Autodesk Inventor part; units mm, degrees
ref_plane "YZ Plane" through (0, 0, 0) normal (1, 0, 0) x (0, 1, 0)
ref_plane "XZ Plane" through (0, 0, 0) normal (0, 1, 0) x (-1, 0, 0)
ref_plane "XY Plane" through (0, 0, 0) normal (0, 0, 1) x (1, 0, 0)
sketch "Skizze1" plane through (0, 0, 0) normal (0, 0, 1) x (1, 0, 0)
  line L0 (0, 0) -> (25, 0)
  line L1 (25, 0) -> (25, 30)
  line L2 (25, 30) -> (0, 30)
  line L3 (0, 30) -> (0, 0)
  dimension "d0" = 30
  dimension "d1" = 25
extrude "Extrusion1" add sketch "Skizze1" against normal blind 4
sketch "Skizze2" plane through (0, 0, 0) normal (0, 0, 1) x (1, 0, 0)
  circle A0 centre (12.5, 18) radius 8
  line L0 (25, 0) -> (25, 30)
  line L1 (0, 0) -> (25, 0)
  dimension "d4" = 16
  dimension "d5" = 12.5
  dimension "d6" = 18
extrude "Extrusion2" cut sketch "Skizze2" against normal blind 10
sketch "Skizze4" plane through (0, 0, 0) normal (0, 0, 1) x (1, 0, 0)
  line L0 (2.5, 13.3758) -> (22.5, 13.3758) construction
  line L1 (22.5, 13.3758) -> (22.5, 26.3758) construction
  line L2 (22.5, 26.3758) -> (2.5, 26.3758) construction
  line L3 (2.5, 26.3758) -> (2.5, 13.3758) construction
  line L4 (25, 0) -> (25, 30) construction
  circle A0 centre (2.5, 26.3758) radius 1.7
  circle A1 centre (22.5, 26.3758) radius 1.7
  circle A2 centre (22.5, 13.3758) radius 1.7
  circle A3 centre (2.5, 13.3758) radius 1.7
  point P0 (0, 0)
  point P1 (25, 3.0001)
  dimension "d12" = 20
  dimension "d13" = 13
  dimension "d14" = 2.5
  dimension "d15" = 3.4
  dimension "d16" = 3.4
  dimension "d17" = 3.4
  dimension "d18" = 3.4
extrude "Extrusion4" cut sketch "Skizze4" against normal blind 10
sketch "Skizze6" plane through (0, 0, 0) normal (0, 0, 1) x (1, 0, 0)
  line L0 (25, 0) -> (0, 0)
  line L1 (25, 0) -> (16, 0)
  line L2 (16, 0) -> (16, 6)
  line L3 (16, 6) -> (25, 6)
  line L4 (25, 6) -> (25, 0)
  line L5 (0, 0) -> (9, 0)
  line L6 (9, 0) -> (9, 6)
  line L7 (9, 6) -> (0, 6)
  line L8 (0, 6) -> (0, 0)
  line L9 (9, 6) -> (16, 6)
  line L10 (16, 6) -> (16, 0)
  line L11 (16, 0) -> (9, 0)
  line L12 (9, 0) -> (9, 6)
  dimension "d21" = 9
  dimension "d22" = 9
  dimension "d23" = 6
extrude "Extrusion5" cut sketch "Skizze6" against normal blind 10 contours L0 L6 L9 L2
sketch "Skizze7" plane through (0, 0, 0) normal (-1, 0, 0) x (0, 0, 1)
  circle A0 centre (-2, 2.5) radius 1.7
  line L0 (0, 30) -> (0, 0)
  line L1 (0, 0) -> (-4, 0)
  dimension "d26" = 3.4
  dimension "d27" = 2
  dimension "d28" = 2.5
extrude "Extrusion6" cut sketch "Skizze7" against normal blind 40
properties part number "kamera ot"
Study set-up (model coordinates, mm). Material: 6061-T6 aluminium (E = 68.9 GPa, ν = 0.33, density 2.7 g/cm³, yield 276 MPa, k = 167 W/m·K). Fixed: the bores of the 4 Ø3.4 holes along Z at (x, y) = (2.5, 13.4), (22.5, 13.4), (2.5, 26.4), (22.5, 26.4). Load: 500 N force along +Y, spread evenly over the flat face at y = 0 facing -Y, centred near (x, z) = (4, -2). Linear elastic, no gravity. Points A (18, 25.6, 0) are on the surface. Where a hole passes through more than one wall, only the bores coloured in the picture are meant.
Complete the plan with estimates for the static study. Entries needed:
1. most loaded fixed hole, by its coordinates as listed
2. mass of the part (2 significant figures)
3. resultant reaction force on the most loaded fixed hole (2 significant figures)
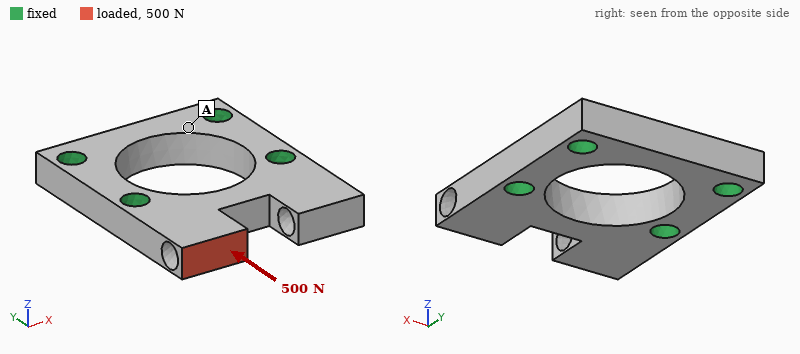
(2.5, 13.4)
4.6 g
460 N
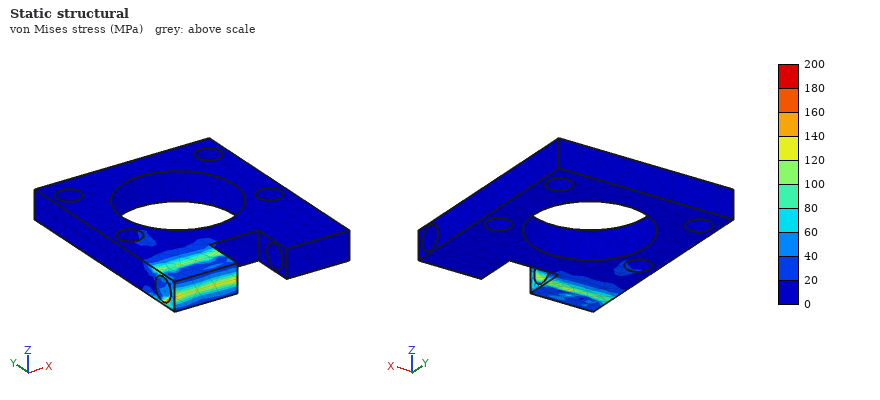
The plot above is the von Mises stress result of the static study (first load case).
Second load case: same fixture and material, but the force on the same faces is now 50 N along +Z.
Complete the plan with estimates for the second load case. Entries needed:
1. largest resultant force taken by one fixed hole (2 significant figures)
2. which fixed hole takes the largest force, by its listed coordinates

46 N
(2.5, 13.4)
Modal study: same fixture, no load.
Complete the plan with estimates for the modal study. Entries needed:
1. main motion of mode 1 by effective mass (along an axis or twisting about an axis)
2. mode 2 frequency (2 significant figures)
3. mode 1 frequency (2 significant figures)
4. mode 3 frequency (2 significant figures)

along Z
23 kHz
20 kHz
40 kHz
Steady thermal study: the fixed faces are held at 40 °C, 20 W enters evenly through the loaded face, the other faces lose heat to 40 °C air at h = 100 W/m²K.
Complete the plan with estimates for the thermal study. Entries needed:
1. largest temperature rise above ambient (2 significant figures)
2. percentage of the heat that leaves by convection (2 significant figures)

78 K
7.3 %
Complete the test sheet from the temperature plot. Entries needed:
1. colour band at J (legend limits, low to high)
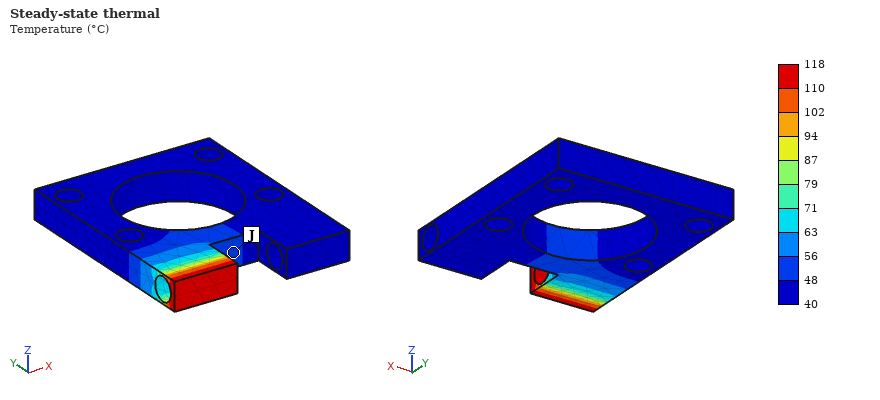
48 to 56 °C
